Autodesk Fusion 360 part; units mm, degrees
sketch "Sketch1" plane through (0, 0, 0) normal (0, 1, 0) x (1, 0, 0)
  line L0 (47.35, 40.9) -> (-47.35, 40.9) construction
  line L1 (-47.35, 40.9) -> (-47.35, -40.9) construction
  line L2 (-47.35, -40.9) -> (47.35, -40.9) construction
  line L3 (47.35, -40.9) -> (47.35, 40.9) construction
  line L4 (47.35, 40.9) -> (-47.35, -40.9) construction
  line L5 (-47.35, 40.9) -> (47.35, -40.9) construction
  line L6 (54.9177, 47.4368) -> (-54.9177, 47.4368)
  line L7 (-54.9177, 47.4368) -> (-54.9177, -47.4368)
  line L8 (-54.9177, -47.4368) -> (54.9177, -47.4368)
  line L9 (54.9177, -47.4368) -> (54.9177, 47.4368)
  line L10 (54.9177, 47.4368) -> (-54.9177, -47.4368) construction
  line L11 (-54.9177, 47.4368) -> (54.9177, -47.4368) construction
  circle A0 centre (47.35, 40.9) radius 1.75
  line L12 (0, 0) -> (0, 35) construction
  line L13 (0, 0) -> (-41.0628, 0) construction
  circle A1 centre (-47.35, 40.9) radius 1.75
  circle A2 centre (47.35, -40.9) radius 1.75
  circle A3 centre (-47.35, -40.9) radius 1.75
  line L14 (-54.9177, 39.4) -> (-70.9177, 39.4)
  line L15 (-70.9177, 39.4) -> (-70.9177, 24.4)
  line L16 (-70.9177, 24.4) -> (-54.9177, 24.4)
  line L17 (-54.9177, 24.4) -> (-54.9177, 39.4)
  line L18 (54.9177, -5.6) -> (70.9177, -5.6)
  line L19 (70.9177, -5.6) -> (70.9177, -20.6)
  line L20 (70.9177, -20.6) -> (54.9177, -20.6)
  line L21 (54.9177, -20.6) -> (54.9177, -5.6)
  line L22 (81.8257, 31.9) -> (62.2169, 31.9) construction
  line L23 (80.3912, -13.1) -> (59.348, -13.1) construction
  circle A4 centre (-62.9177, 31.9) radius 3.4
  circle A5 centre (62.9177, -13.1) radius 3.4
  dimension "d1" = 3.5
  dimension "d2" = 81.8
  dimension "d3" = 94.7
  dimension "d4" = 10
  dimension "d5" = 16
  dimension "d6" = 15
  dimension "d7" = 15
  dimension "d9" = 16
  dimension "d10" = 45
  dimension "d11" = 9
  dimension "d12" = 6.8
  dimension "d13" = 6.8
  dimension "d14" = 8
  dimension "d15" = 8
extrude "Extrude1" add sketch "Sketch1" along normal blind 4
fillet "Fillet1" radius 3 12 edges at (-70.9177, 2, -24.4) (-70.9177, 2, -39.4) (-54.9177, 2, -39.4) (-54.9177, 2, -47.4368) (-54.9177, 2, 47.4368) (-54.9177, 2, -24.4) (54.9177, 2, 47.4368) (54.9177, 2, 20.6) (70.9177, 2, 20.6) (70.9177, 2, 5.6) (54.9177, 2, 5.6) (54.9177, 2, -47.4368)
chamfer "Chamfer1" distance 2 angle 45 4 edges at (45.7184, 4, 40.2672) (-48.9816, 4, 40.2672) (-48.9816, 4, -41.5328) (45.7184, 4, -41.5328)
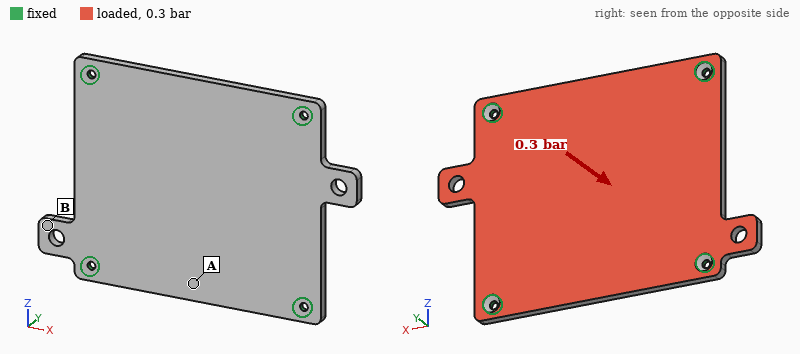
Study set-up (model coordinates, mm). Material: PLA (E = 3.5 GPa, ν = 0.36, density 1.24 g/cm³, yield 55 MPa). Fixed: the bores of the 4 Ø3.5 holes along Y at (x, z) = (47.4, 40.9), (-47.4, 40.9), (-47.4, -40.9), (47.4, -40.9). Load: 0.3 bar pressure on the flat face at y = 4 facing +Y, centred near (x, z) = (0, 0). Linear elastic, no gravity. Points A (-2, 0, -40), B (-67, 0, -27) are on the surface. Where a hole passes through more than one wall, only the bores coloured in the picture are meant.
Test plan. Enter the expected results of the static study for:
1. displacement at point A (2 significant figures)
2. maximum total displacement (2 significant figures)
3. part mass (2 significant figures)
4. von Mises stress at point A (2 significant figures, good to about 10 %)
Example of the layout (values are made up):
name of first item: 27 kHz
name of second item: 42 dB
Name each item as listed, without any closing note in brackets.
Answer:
displacement at point A: 0.69 mm
maximum total displacement: 0.94 mm
part mass: 53 g
von Mises stress at point A: 6.2 MPa
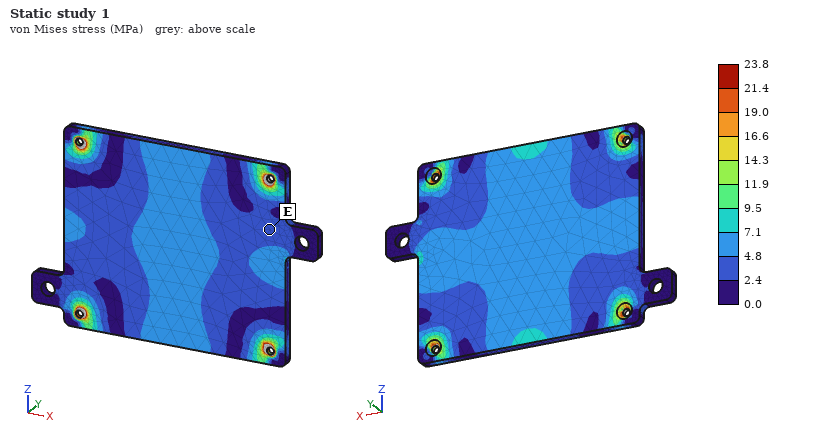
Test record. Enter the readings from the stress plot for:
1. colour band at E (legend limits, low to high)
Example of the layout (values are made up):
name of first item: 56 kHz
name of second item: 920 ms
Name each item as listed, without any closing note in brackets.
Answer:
colour band at E: 2.4 to 4.8 MPa
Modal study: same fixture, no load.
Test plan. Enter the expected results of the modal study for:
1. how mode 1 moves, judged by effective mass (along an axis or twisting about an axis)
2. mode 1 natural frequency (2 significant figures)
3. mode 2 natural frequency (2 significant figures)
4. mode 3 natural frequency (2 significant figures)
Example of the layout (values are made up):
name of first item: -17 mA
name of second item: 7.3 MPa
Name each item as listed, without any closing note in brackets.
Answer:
how mode 1 moves, judged by effective mass: along Y
mode 1 natural frequency: 480 Hz
mode 2 natural frequency: 780 Hz
mode 3 natural frequency: 810 Hz
